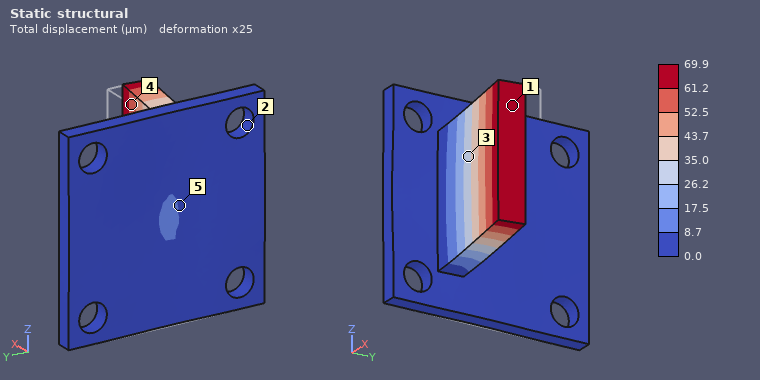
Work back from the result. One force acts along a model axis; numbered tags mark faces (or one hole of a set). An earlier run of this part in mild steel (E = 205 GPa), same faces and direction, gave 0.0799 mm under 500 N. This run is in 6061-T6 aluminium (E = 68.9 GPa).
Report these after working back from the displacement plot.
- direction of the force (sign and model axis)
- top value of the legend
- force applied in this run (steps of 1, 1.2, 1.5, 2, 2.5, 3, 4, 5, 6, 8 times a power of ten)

-Y
69.9 µm
150 N
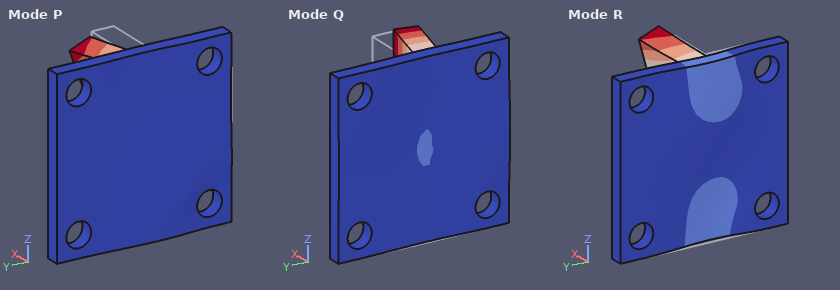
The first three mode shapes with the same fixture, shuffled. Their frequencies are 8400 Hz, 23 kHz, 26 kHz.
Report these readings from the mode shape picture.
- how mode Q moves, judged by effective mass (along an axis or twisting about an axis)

along Y
